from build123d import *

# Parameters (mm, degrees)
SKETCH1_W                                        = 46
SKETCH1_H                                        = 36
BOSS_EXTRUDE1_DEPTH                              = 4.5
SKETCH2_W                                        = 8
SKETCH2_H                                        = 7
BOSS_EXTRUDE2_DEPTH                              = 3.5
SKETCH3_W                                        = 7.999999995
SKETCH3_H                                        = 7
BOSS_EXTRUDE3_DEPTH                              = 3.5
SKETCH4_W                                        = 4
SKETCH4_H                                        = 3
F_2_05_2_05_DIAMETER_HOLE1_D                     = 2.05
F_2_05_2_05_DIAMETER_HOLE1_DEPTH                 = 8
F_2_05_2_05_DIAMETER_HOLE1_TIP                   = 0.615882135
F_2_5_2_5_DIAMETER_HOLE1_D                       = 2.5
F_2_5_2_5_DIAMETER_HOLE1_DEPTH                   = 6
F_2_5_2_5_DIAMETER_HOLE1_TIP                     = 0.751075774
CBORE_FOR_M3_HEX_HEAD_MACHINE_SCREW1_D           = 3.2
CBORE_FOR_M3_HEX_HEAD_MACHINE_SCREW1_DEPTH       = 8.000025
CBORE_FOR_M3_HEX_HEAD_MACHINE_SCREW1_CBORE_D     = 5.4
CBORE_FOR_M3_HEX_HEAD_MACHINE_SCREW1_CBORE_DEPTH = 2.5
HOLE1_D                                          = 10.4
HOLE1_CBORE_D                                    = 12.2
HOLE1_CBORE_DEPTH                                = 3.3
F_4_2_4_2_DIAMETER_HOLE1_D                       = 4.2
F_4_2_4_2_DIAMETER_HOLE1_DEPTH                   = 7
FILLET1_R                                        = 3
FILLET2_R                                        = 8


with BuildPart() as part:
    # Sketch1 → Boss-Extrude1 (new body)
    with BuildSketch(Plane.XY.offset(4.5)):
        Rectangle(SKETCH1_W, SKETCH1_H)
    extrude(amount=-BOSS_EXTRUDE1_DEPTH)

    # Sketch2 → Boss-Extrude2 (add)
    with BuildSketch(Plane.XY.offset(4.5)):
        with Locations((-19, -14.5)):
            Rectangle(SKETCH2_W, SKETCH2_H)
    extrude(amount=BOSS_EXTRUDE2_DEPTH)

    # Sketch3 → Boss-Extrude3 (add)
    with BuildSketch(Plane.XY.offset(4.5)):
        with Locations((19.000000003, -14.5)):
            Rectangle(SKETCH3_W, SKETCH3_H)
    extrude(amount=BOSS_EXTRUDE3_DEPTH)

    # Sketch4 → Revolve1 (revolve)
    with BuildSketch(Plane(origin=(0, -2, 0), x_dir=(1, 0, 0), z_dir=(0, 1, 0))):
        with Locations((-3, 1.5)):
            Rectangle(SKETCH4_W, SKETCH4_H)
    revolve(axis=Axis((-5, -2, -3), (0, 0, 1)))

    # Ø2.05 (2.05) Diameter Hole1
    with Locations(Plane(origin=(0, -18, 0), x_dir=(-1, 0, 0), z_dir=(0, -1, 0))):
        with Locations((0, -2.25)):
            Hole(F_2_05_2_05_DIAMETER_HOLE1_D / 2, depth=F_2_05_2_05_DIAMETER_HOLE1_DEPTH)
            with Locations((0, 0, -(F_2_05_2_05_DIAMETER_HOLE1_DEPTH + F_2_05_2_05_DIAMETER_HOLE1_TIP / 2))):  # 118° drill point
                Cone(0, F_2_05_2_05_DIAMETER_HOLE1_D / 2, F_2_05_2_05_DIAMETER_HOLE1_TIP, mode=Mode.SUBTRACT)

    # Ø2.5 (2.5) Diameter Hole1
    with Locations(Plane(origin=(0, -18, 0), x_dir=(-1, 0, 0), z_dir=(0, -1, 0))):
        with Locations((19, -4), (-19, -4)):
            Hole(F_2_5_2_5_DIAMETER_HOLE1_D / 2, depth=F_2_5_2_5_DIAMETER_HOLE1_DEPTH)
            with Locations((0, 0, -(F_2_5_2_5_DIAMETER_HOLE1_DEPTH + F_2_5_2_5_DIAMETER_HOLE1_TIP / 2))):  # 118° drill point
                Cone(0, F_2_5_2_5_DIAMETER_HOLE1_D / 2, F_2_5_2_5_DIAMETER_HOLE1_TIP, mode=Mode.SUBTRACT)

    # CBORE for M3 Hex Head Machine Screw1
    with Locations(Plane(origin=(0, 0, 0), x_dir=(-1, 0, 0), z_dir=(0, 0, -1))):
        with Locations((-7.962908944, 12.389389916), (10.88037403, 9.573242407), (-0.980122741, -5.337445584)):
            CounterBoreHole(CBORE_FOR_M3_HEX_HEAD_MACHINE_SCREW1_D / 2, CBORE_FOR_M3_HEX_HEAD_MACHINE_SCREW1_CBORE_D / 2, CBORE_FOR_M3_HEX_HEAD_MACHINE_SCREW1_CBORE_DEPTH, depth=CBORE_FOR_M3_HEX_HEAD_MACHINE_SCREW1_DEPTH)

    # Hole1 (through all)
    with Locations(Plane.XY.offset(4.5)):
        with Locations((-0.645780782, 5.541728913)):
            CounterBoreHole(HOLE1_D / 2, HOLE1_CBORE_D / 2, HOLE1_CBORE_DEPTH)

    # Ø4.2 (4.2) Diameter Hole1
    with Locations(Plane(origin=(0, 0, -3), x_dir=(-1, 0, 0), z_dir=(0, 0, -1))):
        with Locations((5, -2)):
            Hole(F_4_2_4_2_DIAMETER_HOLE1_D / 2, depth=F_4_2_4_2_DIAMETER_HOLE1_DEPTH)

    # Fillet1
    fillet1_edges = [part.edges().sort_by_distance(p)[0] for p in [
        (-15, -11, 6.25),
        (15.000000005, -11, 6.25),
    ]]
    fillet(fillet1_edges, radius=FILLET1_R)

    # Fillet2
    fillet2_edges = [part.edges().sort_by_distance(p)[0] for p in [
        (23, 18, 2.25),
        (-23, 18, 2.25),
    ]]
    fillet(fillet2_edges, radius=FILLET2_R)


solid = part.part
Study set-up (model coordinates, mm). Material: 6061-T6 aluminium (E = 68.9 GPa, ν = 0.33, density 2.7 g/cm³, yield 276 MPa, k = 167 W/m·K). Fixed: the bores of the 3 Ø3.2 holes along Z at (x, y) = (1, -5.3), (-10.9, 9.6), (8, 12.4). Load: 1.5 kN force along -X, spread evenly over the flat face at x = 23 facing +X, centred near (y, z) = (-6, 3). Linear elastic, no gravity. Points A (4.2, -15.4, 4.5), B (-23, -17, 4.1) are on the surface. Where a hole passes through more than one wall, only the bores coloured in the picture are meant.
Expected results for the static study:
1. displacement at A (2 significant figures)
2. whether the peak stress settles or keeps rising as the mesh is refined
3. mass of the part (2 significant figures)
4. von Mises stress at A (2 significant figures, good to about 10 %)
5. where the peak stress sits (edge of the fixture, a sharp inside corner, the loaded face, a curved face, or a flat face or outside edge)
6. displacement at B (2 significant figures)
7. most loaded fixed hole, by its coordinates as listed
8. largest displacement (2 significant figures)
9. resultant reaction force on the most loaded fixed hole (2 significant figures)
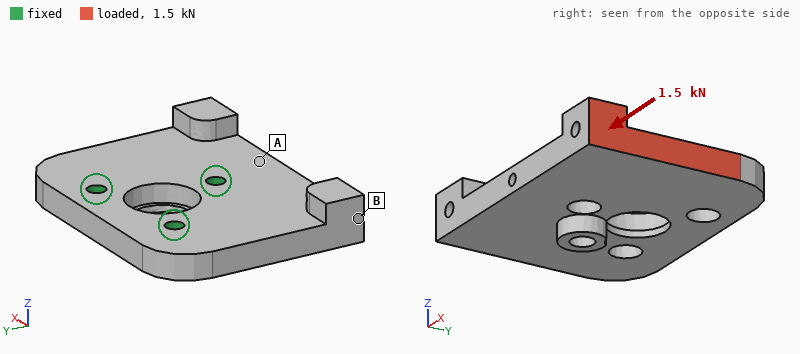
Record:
6.3 µm
keeps rising
19 g
18 MPa
edge of the fixture
7.6 µm
(1, -5.3)
21 µm
1.3 kN
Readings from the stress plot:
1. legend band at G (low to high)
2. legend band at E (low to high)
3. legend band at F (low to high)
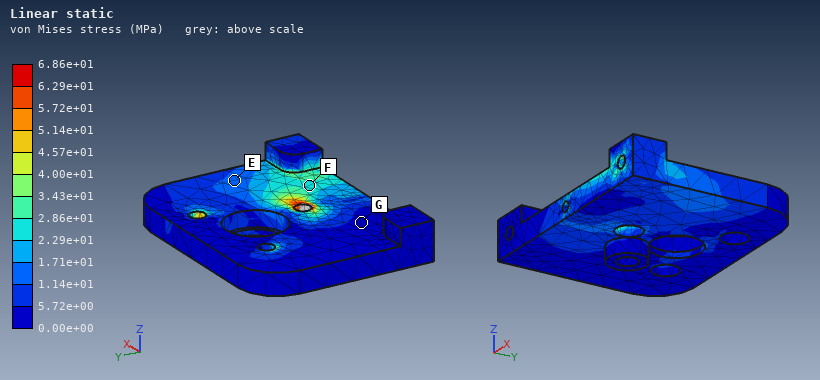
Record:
0.00e+00 to 5.72e+00 MPa
1.14e+01 to 1.71e+01 MPa
2.29e+01 to 2.86e+01 MPa
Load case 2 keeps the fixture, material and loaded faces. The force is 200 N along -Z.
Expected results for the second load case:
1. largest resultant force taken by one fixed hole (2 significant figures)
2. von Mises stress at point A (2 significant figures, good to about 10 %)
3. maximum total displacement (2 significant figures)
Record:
210 N
25 MPa
83 µm
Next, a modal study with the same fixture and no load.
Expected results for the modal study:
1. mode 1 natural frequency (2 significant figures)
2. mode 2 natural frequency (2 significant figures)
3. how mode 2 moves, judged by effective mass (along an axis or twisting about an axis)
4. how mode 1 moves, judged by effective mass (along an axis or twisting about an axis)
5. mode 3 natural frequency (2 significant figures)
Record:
5000 Hz
6300 Hz
along Z
twisting about Y
13 kHz
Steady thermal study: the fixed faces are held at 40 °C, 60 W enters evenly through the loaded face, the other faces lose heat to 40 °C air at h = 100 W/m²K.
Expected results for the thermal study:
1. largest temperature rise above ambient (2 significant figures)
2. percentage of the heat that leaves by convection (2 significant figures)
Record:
68 K
12 %
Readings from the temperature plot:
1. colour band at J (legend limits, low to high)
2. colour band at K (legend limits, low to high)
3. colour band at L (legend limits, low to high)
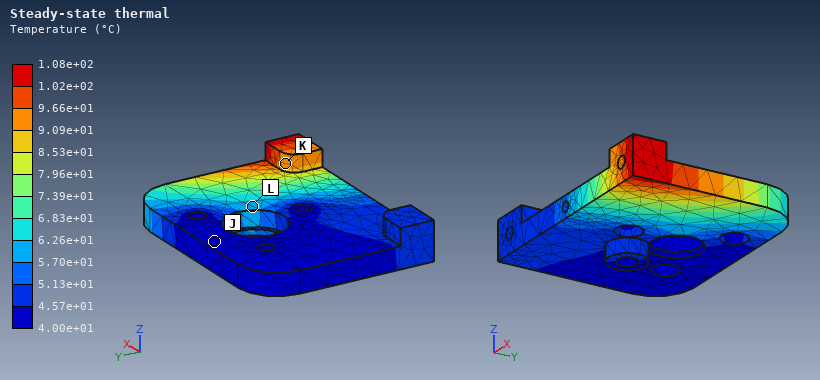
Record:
4.00e+01 to 4.57e+01 °C
9.09e+01 to 9.66e+01 °C
5.70e+01 to 6.26e+01 °C
